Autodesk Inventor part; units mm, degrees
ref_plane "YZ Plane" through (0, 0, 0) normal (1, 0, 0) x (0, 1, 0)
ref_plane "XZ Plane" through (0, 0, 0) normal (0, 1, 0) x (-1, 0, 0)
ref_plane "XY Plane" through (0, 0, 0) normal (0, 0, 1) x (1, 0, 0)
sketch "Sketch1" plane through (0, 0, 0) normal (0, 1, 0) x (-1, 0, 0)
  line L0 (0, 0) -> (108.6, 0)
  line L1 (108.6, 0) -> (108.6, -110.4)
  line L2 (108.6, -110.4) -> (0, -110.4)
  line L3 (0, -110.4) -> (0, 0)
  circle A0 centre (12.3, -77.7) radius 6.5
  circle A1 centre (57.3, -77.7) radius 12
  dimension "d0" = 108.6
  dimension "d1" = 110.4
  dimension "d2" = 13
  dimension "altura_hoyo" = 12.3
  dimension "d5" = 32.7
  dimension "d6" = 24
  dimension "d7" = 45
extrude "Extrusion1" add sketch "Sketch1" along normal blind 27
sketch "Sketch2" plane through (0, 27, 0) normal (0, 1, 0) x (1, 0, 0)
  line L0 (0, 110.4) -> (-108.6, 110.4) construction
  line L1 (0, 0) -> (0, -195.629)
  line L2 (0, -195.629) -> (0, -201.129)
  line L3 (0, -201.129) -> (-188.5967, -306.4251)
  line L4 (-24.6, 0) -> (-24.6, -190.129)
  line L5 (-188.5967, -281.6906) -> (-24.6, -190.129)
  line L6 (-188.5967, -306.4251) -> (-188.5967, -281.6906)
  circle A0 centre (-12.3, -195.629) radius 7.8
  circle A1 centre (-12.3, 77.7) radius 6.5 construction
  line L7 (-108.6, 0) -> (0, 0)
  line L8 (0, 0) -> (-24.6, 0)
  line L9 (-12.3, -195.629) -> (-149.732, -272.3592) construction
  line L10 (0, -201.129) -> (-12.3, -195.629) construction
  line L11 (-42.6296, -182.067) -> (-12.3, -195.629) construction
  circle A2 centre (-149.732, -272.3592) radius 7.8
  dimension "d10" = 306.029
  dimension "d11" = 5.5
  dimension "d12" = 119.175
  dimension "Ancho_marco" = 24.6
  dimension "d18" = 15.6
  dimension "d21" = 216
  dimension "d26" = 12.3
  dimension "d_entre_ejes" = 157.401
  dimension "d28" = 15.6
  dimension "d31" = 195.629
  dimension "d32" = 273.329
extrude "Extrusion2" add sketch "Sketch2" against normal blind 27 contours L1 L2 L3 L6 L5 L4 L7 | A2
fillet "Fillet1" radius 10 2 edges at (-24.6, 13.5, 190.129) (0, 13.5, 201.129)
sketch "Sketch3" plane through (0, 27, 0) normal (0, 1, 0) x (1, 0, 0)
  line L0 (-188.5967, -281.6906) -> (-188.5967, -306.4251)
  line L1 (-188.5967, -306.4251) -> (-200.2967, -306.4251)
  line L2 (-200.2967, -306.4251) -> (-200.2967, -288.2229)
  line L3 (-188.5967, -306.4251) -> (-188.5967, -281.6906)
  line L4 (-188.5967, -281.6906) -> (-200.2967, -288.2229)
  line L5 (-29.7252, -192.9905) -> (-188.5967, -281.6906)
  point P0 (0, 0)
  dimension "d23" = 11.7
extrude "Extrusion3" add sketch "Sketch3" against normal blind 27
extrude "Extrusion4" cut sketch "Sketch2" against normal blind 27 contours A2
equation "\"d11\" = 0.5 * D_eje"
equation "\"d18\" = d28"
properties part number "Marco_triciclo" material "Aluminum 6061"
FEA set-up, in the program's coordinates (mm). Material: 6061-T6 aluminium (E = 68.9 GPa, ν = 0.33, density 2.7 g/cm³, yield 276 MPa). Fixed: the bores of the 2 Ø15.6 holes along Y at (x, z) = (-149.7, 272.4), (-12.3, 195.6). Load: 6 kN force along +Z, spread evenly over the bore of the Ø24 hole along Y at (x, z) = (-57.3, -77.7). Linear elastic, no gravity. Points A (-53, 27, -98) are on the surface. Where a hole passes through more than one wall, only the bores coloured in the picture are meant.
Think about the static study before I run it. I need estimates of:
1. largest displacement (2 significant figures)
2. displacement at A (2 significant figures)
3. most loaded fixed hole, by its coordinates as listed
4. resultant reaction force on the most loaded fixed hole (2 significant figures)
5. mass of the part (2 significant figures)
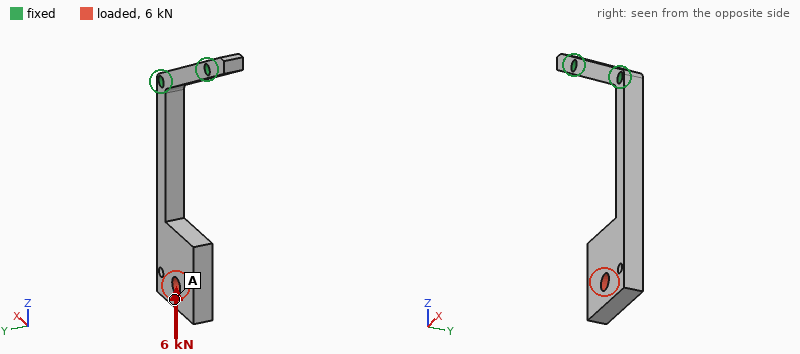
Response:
5.4 mm
4.6 mm
(-12.3, 195.6)
5.7 kN
1.5 kg
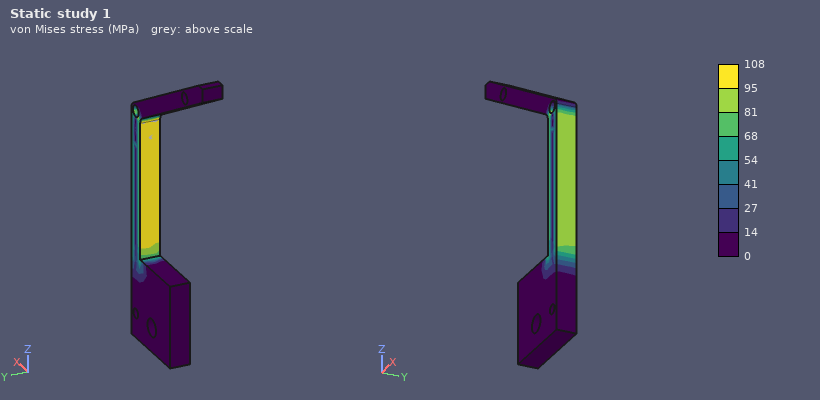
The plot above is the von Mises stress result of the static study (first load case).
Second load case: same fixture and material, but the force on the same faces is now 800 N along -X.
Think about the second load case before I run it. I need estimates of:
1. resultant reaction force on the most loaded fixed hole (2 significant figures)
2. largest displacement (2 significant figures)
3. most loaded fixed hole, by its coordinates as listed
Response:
670 N
2.9 mm
(-12.3, 195.6)
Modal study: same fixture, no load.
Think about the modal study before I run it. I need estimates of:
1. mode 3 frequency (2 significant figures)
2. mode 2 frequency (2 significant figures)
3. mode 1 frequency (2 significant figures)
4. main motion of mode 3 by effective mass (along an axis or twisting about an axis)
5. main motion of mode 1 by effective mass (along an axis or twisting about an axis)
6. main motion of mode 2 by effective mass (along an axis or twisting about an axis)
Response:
480 Hz
120 Hz
110 Hz
twisting about Z
along X
along Y
